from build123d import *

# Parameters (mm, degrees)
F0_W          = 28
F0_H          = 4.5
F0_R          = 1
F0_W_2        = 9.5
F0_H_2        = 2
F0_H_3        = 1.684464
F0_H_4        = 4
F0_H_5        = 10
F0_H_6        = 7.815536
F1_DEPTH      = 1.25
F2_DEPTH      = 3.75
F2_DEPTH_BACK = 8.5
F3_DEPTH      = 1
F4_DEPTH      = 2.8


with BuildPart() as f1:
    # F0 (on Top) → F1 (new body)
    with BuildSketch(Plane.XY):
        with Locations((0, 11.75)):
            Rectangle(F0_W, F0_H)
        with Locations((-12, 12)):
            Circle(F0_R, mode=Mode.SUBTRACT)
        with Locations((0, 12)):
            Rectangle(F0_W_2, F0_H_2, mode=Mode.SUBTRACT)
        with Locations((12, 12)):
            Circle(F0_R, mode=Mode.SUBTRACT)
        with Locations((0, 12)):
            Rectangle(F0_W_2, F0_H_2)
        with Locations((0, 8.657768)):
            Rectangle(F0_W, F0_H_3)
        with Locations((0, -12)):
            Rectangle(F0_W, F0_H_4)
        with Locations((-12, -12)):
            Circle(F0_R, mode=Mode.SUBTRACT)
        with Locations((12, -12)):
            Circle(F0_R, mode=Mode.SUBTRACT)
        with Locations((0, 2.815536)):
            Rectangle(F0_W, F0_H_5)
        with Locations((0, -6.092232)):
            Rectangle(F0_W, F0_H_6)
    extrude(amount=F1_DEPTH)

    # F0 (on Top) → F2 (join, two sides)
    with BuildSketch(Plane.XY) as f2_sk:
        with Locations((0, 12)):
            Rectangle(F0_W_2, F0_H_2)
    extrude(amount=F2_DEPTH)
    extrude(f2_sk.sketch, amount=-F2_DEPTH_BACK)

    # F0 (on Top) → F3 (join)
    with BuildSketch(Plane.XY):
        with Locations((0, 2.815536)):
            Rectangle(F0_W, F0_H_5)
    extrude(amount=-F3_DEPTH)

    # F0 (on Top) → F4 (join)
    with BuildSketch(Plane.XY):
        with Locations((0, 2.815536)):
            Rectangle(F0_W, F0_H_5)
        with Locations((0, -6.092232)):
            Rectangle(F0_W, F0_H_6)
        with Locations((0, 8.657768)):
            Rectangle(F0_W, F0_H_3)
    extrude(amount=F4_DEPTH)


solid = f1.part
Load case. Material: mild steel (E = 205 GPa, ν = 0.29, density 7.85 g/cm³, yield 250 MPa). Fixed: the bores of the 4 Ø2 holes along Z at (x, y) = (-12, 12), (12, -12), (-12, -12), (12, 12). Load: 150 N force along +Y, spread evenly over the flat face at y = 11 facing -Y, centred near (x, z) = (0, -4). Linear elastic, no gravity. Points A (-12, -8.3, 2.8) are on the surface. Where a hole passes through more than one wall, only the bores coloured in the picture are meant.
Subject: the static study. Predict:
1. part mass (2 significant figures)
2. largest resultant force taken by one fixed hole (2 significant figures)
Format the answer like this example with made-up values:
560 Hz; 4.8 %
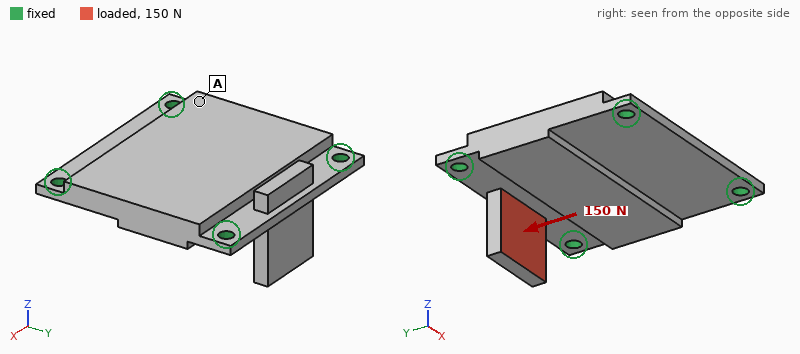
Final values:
18 g; 62 N
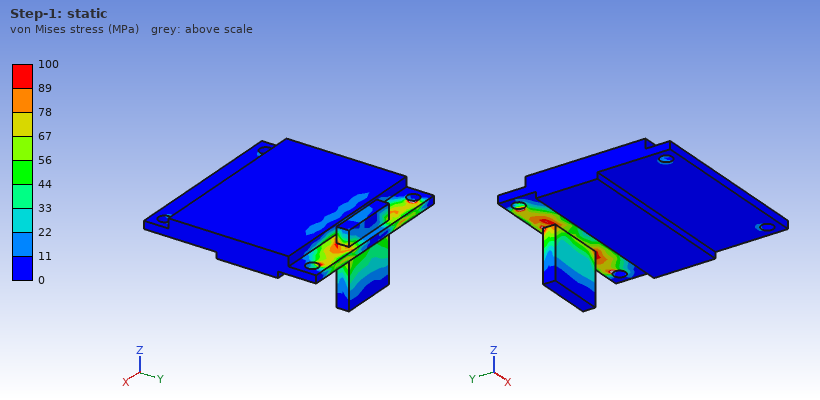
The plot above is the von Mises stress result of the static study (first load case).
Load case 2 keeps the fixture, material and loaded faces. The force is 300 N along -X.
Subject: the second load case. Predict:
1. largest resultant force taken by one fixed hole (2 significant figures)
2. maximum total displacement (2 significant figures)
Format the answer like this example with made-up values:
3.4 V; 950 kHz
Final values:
140 N; 14 µm
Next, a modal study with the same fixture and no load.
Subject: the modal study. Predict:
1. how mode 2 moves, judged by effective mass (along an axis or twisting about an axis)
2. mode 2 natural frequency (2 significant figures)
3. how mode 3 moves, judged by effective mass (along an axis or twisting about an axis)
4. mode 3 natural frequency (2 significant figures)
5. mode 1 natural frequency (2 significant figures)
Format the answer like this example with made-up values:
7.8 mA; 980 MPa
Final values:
along Z; 11 kHz; twisting about X; 19 kHz; 10 kHz
